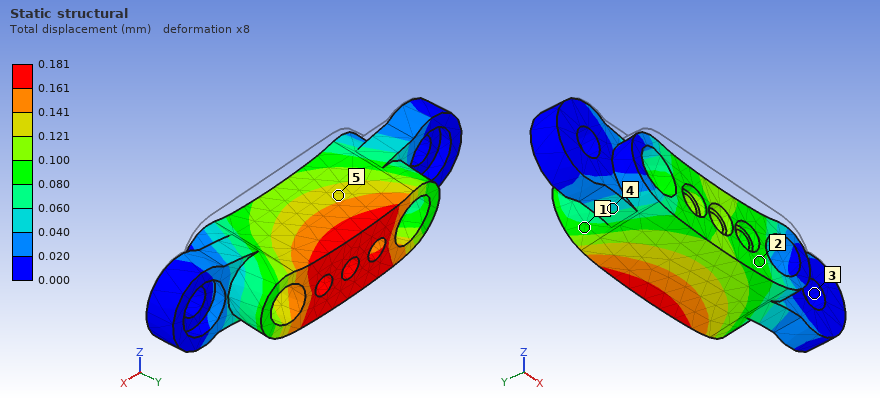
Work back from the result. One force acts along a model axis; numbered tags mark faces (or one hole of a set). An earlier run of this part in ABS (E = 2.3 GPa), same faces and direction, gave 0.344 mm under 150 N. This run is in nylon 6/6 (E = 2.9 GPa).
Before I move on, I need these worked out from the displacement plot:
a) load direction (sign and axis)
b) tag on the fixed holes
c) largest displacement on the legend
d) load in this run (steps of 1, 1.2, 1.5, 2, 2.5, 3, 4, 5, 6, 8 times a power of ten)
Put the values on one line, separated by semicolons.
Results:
-Z; 3; 0.181 mm; 100 N
